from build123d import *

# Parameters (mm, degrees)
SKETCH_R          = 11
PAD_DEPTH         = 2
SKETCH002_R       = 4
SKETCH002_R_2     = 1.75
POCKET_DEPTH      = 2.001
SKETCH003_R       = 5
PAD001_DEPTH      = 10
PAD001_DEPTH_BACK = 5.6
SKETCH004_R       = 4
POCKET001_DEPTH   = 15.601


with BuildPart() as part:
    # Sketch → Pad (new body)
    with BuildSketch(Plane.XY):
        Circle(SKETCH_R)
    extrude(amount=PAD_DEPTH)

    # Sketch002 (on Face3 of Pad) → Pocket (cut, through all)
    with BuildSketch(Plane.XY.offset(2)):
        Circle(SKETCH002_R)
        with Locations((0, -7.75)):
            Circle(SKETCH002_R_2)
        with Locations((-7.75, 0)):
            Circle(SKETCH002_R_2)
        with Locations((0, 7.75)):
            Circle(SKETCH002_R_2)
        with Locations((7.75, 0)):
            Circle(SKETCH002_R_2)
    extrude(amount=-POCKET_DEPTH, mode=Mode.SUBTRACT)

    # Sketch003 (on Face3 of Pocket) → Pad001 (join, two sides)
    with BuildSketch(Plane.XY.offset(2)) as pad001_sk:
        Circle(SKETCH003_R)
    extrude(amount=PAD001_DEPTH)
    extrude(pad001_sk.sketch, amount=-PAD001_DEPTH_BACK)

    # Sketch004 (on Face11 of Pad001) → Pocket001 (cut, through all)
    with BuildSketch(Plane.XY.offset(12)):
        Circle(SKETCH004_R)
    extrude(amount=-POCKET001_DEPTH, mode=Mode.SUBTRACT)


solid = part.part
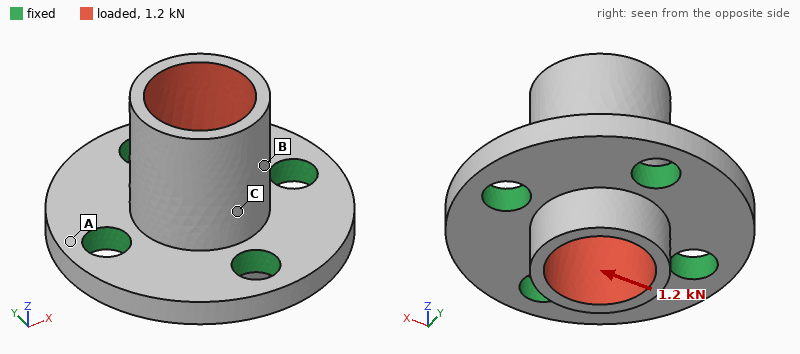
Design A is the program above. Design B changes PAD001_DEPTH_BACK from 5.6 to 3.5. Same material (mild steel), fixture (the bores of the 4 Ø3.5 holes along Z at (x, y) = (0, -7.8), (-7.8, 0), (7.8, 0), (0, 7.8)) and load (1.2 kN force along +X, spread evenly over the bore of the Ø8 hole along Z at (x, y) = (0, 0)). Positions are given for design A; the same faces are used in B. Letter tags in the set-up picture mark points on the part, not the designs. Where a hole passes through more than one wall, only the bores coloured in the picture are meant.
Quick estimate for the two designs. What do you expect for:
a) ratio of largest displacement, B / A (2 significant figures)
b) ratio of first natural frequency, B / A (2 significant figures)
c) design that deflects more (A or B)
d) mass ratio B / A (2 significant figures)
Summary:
1.2
1.00
B
0.94
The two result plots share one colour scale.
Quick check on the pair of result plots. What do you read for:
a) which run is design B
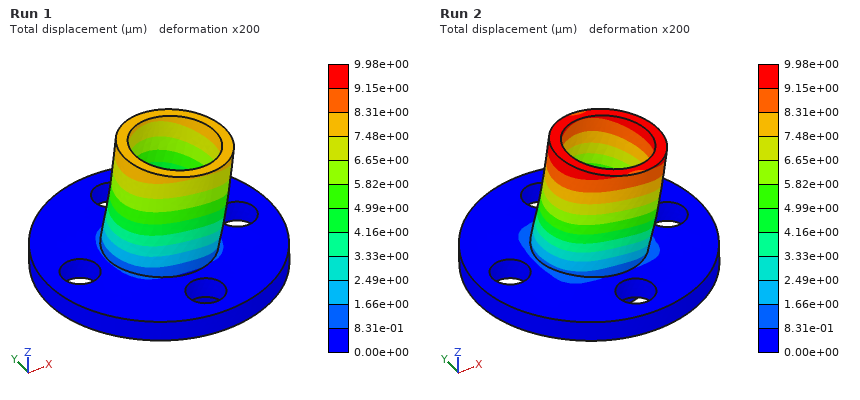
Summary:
Run 2
